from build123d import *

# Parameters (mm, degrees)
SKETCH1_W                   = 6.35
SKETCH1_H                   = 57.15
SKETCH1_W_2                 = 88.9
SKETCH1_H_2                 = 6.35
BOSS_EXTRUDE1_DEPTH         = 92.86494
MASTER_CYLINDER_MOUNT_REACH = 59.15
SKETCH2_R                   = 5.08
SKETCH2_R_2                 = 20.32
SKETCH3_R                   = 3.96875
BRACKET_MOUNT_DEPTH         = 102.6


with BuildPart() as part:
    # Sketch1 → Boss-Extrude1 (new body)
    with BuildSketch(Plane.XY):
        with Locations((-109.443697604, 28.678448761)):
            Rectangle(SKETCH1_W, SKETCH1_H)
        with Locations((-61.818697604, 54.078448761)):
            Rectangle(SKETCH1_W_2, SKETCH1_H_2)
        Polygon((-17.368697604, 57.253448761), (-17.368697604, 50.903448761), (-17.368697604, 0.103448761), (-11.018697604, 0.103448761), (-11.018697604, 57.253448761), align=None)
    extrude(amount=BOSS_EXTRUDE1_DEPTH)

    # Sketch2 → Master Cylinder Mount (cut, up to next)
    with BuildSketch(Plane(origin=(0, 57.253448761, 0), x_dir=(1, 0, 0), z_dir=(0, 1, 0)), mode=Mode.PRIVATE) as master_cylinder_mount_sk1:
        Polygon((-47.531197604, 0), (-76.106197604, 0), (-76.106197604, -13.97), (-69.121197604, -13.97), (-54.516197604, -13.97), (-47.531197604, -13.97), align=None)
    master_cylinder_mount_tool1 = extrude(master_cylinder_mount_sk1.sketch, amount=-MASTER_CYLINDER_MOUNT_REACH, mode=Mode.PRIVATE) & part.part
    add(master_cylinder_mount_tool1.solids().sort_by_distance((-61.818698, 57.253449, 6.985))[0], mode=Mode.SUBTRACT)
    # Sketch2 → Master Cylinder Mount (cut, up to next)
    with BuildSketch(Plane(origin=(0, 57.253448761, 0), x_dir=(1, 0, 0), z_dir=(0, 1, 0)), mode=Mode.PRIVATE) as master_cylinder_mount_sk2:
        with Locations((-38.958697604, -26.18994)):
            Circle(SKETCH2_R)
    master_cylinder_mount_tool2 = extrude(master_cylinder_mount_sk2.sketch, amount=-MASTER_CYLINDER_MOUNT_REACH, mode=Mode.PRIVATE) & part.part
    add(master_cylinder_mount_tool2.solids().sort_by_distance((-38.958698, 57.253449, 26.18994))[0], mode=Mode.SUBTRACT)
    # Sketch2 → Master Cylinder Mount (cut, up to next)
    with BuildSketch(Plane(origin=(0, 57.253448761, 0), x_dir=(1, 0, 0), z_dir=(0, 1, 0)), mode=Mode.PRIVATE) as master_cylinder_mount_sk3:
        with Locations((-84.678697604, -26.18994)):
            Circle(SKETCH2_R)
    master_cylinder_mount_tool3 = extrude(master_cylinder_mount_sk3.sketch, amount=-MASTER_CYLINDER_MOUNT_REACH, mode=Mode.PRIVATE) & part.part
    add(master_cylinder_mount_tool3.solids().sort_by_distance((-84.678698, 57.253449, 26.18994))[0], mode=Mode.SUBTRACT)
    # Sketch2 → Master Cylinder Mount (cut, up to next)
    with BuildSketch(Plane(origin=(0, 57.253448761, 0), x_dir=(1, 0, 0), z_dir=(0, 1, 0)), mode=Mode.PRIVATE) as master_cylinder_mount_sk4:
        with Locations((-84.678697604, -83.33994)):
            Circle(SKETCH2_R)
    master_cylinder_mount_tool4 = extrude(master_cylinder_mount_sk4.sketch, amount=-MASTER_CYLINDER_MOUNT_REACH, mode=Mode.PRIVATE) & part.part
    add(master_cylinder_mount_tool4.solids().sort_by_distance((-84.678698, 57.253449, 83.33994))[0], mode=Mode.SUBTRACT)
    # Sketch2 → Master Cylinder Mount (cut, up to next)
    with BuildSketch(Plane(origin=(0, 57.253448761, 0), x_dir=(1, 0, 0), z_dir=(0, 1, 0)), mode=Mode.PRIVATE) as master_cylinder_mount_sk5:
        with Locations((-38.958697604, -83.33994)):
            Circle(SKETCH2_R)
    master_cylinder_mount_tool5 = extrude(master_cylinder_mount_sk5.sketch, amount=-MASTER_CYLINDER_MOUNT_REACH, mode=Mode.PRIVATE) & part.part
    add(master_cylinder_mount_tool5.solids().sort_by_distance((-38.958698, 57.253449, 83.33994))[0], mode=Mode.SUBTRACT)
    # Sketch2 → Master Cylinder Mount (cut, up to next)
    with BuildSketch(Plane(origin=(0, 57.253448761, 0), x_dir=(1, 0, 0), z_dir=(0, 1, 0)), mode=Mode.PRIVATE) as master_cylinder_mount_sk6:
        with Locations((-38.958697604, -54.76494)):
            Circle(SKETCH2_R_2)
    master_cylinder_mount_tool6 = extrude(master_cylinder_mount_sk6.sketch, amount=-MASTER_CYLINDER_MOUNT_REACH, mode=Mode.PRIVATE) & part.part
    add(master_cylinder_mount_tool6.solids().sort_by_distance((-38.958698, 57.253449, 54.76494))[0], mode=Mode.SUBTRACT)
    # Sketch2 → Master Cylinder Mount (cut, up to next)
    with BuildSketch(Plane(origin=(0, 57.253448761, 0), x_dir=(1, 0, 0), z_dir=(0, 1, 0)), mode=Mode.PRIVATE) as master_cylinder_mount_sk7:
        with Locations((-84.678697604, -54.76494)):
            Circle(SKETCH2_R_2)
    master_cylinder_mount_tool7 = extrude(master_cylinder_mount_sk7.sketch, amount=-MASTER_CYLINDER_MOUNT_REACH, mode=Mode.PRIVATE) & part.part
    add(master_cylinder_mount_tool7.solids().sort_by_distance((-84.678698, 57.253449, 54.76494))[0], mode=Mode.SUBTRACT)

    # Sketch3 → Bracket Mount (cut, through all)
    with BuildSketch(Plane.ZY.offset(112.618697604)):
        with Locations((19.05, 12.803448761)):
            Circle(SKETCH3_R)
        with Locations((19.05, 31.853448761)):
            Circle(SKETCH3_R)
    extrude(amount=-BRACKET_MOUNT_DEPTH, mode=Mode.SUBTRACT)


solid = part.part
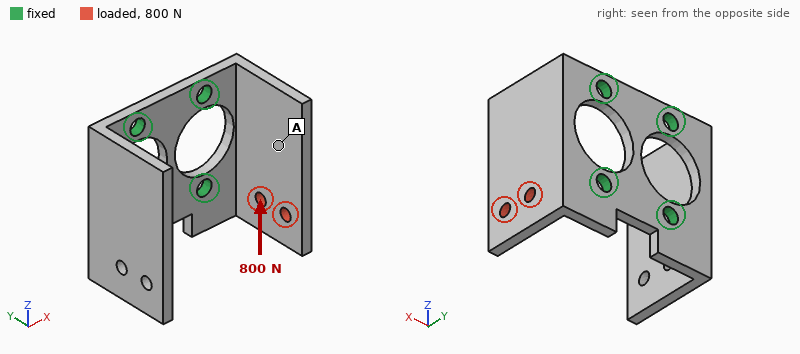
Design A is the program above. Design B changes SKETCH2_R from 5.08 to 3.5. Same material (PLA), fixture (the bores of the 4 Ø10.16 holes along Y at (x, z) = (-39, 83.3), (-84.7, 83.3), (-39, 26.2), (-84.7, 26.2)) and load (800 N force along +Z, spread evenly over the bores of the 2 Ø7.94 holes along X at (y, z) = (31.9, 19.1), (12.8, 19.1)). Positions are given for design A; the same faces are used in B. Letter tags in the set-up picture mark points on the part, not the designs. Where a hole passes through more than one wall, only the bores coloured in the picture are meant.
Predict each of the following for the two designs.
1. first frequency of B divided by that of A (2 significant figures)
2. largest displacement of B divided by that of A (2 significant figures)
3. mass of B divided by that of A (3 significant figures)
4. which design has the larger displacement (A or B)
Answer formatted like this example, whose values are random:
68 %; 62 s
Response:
0.94; 1.2; 1.01; B
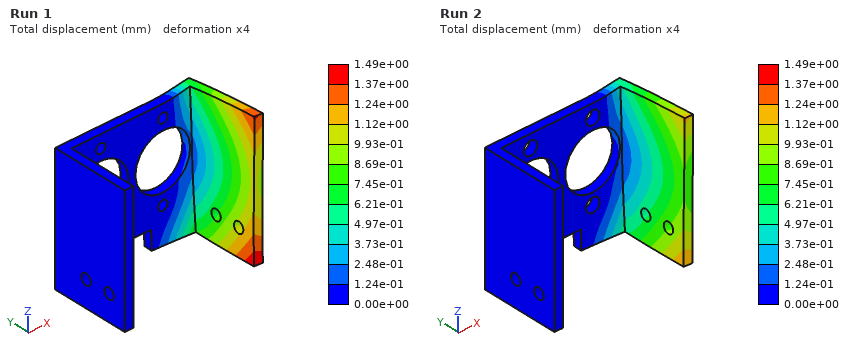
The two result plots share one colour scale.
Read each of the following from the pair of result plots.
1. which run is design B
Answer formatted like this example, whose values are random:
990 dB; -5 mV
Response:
Run 1
